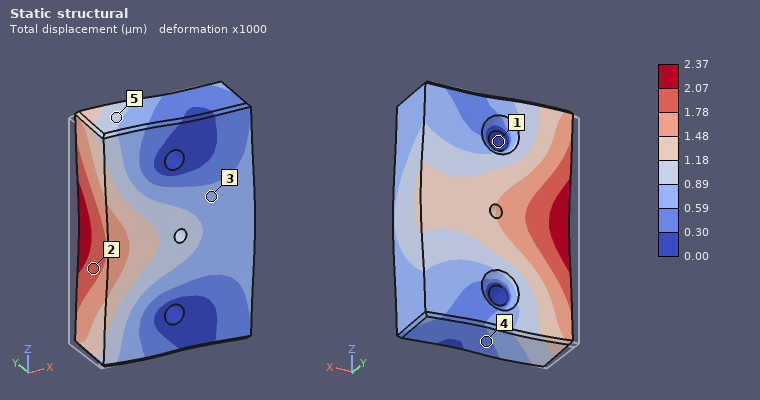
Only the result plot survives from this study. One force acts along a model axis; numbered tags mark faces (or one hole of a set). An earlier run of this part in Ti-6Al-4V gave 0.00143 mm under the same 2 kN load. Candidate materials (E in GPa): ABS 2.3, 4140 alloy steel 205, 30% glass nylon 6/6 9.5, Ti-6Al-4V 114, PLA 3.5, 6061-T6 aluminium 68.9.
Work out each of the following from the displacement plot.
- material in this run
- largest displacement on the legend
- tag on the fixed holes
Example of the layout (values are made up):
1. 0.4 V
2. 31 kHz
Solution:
1. 6061-T6 aluminium
2. 2.37 µm
3. 1
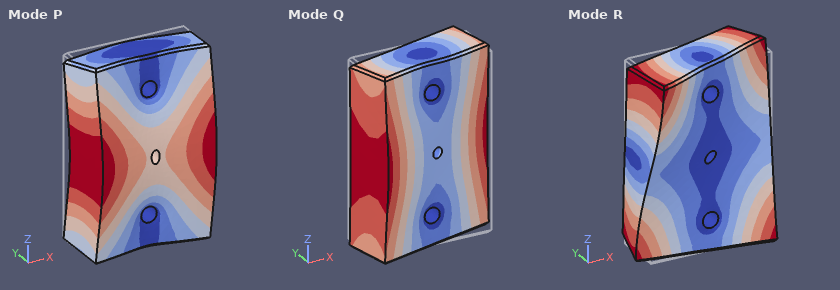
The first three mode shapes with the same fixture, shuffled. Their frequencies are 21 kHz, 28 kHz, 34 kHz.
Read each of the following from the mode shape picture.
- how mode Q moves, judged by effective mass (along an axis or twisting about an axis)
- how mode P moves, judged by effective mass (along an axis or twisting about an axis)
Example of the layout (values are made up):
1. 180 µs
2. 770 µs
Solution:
1. twisting about Z
2. along Y
